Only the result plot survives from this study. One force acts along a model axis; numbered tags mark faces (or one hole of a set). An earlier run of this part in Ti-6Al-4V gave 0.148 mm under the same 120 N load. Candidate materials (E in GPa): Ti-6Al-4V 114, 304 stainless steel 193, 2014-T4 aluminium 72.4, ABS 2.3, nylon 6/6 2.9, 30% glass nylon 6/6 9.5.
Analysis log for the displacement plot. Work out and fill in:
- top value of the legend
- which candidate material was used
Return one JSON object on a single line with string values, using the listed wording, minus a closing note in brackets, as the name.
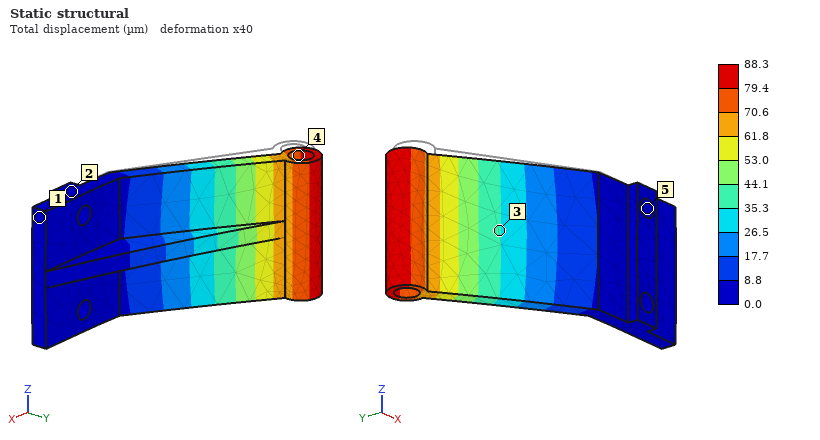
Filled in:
{"top value of the legend": "88.3 µm", "which candidate material was used": "304 stainless steel"}
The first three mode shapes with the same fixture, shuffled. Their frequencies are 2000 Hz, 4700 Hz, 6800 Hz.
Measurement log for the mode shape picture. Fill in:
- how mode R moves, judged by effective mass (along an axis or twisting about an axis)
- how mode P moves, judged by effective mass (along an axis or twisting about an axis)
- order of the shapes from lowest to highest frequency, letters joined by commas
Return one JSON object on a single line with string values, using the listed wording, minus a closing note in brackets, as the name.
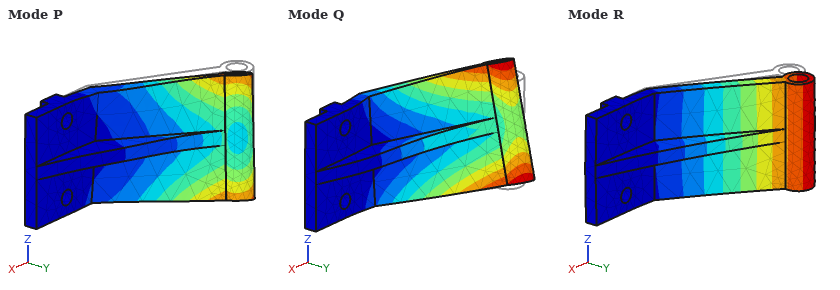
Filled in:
{"how mode R moves, judged by effective mass": "along Y", "how mode P moves, judged by effective mass": "along Z", "order of the shapes from lowest to highest frequency, letters joined by commas": "R, Q, P"}
